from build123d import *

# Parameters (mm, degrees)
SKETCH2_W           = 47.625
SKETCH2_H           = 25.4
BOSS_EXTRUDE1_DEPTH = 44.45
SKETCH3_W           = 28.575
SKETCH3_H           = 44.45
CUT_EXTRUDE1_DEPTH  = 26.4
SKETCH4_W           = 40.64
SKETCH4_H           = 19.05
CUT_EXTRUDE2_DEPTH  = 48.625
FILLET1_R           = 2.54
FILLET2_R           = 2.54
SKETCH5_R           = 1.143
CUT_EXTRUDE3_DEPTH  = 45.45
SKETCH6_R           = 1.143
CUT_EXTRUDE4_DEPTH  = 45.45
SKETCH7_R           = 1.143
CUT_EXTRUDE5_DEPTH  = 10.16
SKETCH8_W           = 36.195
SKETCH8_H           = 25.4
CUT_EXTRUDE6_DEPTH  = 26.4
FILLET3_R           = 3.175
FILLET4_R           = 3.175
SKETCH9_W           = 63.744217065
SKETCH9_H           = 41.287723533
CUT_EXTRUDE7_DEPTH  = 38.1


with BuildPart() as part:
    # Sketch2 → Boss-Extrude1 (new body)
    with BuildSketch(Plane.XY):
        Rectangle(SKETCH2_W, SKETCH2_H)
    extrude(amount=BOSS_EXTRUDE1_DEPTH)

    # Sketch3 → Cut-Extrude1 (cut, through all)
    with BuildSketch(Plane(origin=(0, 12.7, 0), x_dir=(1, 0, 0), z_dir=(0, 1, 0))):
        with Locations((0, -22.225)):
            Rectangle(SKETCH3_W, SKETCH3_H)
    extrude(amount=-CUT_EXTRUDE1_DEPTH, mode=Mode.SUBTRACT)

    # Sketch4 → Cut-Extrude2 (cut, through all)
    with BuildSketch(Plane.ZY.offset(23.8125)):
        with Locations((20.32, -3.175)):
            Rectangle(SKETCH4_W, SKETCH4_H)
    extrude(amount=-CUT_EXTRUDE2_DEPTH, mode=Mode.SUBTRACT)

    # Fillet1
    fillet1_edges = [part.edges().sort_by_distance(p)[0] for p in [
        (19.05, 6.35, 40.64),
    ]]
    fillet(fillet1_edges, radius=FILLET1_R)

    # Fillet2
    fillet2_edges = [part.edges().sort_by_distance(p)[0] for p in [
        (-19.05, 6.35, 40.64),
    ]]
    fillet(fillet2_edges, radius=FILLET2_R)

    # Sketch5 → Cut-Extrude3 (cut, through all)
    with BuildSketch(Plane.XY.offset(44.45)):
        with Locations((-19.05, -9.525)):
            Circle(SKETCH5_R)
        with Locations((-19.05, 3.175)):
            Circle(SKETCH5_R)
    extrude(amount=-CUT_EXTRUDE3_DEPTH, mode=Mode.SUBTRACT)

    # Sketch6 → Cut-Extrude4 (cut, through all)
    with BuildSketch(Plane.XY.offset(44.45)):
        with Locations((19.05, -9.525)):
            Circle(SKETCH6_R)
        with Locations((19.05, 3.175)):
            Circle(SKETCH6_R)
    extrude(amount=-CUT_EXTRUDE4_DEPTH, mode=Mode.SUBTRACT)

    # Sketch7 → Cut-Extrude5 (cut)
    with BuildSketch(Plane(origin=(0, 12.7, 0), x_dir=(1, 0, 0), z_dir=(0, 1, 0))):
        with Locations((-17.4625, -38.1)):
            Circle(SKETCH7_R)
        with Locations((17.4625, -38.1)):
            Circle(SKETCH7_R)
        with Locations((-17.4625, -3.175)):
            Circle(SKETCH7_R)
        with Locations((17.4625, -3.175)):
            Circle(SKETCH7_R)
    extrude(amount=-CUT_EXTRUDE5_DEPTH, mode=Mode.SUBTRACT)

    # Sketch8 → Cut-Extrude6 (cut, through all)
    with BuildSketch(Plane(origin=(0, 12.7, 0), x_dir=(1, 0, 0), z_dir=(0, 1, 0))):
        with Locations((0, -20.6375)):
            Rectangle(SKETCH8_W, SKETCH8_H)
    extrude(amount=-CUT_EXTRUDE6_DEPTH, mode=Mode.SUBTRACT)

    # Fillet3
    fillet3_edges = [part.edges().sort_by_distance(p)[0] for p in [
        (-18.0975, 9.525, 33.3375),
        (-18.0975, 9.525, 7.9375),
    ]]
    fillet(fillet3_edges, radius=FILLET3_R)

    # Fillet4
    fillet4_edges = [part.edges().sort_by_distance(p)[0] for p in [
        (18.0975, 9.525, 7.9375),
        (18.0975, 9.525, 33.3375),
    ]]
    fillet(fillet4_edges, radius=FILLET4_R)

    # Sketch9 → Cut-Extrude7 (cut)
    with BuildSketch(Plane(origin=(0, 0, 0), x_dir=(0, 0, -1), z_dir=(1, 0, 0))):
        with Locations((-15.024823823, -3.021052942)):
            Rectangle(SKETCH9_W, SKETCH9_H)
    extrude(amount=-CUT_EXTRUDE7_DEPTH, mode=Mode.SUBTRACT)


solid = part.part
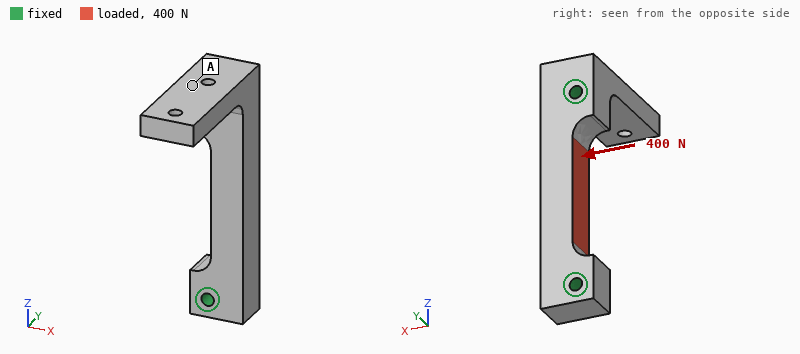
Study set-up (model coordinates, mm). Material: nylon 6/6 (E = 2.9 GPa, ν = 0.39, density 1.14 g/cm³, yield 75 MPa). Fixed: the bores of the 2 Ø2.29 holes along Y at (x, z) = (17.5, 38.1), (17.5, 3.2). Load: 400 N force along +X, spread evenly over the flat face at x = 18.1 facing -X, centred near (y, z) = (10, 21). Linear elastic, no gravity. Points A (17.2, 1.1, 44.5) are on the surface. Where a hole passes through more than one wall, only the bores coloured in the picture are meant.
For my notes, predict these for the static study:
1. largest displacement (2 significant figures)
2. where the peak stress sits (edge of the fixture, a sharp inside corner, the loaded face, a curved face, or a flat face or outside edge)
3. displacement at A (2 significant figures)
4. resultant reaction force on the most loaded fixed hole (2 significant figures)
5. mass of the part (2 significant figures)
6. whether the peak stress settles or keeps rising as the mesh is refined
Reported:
0.25 mm
edge of the fixture
0.042 mm
300 N
3.1 g
keeps rising
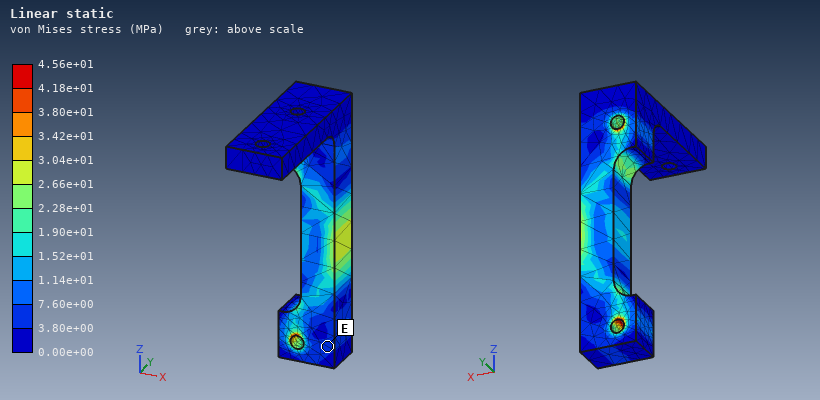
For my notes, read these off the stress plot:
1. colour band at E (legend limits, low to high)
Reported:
3.80e+00 to 7.60e+00 MPa
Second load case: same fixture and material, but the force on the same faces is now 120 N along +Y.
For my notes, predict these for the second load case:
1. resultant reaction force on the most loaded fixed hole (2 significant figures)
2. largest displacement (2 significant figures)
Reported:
60 N
0.10 mm
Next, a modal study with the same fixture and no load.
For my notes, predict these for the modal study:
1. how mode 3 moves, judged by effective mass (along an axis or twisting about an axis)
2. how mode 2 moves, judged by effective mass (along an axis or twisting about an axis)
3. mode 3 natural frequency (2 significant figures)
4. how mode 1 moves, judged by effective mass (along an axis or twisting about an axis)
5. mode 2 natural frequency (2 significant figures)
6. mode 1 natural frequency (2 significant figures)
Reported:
along Y
along X
7000 Hz
along Z
3500 Hz
2300 Hz
